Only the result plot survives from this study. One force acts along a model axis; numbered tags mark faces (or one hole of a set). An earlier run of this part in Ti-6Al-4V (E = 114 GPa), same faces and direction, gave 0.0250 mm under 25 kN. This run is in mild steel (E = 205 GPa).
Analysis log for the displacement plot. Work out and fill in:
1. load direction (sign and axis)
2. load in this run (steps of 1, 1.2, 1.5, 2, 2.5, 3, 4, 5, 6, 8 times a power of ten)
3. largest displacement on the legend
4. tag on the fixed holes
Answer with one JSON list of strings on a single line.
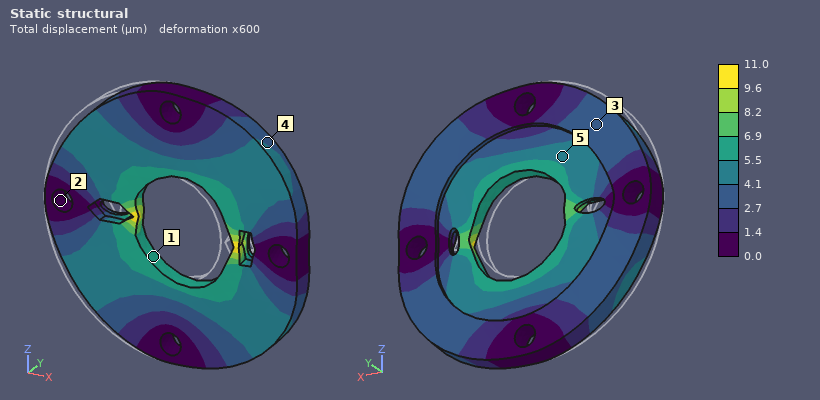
["+X", "20 kN", "11.0 µm", "2"]
